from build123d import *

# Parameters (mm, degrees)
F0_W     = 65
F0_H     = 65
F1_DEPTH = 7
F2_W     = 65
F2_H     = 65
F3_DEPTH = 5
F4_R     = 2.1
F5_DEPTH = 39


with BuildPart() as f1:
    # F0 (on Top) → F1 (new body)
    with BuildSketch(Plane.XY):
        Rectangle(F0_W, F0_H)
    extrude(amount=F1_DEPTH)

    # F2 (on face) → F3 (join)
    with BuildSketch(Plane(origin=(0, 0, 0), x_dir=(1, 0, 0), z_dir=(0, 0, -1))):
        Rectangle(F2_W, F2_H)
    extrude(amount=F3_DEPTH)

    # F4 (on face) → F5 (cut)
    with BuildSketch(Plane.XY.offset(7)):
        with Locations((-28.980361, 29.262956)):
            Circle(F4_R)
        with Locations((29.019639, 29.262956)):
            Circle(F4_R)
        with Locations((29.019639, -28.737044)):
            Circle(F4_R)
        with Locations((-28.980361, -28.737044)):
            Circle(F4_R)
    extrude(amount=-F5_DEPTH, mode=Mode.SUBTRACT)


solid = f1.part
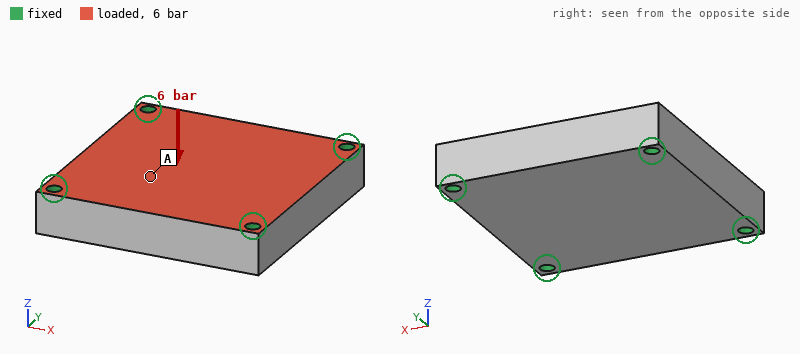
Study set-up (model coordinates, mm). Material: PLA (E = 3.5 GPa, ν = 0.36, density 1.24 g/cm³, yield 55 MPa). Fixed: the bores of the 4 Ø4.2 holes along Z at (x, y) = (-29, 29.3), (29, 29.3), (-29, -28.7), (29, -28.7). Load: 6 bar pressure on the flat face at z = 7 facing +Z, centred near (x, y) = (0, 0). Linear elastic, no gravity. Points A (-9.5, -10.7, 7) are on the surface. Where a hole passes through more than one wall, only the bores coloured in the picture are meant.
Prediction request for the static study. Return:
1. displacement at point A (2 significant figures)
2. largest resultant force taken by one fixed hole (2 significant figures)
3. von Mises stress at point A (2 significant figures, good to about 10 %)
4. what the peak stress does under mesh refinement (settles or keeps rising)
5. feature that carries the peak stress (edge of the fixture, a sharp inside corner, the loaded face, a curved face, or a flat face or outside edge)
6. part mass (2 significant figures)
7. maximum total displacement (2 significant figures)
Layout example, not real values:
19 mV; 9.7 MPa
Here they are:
0.12 mm; 630 N; 3.8 MPa; keeps rising; edge of the fixture; 62 g; 0.14 mm
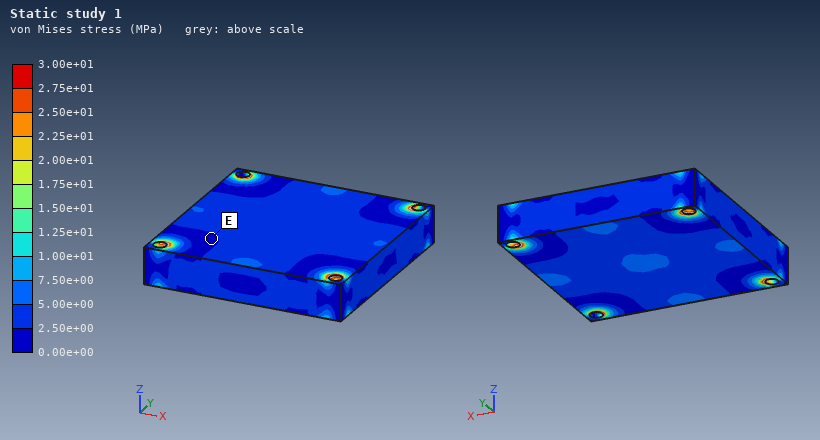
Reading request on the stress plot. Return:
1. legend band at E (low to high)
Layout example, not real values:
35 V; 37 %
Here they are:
0.00e+00 to 2.50e+00 MPa
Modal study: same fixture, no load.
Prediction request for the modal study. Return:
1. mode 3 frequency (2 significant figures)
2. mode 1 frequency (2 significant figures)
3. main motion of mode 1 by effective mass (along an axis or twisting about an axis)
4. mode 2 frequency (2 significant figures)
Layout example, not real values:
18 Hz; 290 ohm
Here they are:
5100 Hz; 3100 Hz; along Z; 5100 Hz
